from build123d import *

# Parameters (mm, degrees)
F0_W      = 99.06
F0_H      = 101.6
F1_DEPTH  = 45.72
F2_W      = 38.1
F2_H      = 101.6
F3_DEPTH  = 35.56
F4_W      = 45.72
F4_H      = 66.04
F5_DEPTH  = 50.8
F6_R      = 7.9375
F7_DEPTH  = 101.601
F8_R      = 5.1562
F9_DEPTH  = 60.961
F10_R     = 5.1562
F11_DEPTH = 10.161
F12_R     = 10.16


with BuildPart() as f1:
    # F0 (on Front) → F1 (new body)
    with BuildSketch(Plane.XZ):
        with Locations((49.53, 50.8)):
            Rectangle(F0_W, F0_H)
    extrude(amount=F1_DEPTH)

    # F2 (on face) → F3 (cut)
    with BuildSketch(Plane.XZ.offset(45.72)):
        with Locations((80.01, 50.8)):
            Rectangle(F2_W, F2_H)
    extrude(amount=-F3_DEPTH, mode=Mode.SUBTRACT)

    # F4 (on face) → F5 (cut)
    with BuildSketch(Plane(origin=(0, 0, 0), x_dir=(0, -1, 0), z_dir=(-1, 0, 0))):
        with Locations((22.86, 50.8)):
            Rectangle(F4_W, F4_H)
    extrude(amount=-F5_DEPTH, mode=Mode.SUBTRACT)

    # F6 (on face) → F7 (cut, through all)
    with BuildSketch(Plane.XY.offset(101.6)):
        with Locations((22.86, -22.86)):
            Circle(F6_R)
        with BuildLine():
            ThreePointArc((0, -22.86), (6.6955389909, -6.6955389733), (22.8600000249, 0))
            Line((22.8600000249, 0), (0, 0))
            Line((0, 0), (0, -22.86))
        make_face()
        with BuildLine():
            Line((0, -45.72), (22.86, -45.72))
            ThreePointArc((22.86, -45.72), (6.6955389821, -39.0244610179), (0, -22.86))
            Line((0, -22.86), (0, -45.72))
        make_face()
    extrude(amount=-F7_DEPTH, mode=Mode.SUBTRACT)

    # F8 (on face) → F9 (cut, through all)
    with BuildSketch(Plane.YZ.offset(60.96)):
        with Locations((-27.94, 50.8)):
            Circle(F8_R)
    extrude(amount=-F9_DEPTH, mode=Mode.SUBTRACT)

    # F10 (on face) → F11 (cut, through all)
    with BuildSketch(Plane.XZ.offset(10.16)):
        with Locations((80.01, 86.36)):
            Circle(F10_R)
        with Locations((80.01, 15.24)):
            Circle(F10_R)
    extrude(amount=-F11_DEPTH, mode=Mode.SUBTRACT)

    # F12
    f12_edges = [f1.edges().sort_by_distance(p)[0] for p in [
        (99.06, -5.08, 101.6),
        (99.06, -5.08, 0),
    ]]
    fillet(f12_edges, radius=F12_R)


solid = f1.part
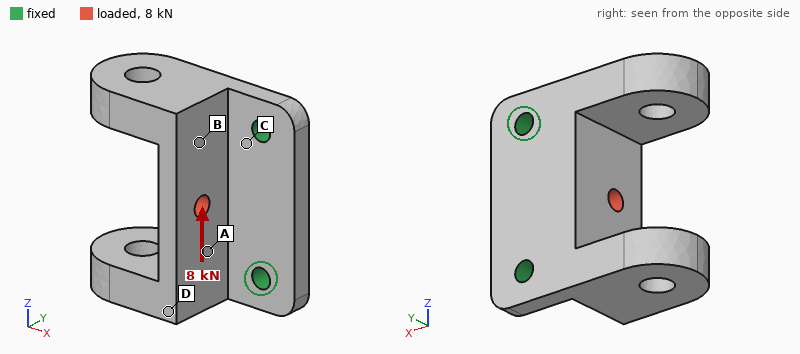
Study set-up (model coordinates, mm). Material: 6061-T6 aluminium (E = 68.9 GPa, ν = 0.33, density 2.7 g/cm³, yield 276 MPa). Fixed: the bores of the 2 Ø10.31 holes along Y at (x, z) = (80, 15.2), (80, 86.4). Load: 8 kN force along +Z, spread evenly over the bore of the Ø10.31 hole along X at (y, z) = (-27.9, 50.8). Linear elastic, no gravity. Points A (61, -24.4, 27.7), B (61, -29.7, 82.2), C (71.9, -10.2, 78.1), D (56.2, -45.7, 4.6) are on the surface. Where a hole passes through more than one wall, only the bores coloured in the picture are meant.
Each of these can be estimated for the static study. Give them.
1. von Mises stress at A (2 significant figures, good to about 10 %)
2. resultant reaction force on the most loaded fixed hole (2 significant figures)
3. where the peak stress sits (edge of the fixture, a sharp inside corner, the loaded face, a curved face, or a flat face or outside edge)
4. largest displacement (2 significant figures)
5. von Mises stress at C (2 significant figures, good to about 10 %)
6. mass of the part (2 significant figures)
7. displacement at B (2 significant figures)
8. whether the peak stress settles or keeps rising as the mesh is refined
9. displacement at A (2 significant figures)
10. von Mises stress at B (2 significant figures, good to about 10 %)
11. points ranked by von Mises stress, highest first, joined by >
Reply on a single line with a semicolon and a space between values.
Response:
25 MPa; 5.2 kN; edge of the fixture; 94 µm; 34 MPa; 410 g; 42 µm; keeps rising; 34 µm; 17 MPa; C > A > B > D
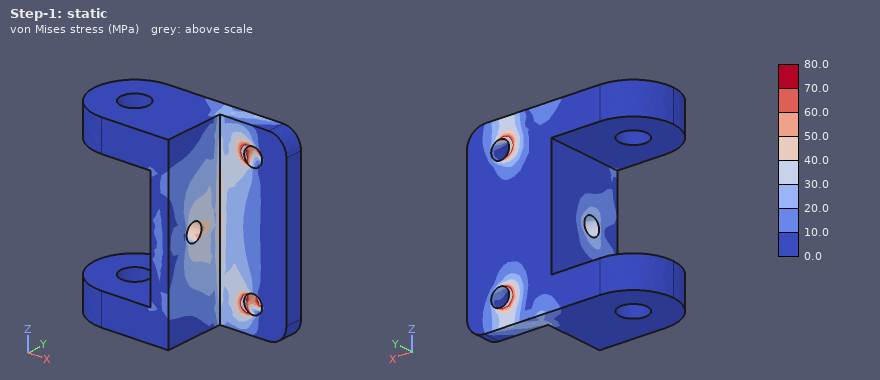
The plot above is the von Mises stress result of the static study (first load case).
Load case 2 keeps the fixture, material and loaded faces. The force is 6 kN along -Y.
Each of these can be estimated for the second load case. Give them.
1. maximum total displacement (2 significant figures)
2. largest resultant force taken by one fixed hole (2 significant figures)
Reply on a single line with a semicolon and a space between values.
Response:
0.24 mm; 3.0 kN
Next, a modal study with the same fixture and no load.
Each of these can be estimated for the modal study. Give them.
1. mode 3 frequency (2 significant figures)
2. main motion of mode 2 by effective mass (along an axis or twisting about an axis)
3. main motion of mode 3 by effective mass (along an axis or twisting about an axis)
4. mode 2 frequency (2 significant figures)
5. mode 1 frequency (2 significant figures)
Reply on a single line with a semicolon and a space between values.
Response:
2800 Hz; twisting about X; along Z; 1500 Hz; 1100 Hz
